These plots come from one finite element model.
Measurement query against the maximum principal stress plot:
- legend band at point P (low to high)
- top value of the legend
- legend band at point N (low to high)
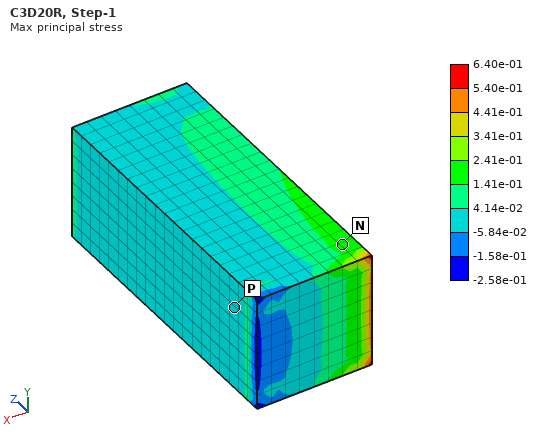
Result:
-5.84e-02 to 4.14e-02
6.40e-01
1.41e-01 to 2.41e-01
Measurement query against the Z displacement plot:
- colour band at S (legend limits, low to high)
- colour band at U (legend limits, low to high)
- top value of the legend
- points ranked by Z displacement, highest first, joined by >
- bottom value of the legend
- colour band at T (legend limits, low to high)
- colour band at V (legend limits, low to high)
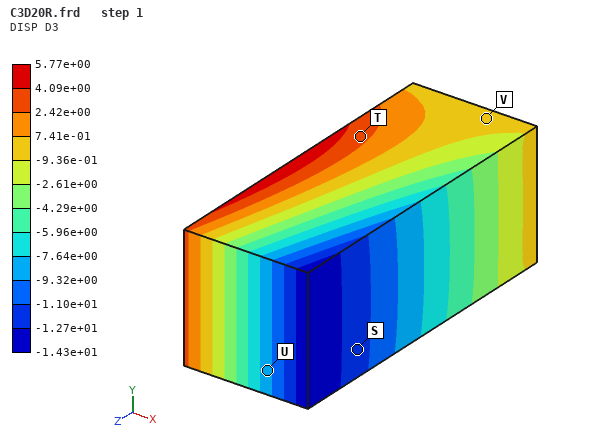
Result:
-1.27e+01 to -1.10e+01
-9.32e+00 to -7.64e+00
5.77e+00
T > V > U > S
-1.43e+01
2.42e+00 to 4.09e+00
-9.36e-01 to 7.41e-01
